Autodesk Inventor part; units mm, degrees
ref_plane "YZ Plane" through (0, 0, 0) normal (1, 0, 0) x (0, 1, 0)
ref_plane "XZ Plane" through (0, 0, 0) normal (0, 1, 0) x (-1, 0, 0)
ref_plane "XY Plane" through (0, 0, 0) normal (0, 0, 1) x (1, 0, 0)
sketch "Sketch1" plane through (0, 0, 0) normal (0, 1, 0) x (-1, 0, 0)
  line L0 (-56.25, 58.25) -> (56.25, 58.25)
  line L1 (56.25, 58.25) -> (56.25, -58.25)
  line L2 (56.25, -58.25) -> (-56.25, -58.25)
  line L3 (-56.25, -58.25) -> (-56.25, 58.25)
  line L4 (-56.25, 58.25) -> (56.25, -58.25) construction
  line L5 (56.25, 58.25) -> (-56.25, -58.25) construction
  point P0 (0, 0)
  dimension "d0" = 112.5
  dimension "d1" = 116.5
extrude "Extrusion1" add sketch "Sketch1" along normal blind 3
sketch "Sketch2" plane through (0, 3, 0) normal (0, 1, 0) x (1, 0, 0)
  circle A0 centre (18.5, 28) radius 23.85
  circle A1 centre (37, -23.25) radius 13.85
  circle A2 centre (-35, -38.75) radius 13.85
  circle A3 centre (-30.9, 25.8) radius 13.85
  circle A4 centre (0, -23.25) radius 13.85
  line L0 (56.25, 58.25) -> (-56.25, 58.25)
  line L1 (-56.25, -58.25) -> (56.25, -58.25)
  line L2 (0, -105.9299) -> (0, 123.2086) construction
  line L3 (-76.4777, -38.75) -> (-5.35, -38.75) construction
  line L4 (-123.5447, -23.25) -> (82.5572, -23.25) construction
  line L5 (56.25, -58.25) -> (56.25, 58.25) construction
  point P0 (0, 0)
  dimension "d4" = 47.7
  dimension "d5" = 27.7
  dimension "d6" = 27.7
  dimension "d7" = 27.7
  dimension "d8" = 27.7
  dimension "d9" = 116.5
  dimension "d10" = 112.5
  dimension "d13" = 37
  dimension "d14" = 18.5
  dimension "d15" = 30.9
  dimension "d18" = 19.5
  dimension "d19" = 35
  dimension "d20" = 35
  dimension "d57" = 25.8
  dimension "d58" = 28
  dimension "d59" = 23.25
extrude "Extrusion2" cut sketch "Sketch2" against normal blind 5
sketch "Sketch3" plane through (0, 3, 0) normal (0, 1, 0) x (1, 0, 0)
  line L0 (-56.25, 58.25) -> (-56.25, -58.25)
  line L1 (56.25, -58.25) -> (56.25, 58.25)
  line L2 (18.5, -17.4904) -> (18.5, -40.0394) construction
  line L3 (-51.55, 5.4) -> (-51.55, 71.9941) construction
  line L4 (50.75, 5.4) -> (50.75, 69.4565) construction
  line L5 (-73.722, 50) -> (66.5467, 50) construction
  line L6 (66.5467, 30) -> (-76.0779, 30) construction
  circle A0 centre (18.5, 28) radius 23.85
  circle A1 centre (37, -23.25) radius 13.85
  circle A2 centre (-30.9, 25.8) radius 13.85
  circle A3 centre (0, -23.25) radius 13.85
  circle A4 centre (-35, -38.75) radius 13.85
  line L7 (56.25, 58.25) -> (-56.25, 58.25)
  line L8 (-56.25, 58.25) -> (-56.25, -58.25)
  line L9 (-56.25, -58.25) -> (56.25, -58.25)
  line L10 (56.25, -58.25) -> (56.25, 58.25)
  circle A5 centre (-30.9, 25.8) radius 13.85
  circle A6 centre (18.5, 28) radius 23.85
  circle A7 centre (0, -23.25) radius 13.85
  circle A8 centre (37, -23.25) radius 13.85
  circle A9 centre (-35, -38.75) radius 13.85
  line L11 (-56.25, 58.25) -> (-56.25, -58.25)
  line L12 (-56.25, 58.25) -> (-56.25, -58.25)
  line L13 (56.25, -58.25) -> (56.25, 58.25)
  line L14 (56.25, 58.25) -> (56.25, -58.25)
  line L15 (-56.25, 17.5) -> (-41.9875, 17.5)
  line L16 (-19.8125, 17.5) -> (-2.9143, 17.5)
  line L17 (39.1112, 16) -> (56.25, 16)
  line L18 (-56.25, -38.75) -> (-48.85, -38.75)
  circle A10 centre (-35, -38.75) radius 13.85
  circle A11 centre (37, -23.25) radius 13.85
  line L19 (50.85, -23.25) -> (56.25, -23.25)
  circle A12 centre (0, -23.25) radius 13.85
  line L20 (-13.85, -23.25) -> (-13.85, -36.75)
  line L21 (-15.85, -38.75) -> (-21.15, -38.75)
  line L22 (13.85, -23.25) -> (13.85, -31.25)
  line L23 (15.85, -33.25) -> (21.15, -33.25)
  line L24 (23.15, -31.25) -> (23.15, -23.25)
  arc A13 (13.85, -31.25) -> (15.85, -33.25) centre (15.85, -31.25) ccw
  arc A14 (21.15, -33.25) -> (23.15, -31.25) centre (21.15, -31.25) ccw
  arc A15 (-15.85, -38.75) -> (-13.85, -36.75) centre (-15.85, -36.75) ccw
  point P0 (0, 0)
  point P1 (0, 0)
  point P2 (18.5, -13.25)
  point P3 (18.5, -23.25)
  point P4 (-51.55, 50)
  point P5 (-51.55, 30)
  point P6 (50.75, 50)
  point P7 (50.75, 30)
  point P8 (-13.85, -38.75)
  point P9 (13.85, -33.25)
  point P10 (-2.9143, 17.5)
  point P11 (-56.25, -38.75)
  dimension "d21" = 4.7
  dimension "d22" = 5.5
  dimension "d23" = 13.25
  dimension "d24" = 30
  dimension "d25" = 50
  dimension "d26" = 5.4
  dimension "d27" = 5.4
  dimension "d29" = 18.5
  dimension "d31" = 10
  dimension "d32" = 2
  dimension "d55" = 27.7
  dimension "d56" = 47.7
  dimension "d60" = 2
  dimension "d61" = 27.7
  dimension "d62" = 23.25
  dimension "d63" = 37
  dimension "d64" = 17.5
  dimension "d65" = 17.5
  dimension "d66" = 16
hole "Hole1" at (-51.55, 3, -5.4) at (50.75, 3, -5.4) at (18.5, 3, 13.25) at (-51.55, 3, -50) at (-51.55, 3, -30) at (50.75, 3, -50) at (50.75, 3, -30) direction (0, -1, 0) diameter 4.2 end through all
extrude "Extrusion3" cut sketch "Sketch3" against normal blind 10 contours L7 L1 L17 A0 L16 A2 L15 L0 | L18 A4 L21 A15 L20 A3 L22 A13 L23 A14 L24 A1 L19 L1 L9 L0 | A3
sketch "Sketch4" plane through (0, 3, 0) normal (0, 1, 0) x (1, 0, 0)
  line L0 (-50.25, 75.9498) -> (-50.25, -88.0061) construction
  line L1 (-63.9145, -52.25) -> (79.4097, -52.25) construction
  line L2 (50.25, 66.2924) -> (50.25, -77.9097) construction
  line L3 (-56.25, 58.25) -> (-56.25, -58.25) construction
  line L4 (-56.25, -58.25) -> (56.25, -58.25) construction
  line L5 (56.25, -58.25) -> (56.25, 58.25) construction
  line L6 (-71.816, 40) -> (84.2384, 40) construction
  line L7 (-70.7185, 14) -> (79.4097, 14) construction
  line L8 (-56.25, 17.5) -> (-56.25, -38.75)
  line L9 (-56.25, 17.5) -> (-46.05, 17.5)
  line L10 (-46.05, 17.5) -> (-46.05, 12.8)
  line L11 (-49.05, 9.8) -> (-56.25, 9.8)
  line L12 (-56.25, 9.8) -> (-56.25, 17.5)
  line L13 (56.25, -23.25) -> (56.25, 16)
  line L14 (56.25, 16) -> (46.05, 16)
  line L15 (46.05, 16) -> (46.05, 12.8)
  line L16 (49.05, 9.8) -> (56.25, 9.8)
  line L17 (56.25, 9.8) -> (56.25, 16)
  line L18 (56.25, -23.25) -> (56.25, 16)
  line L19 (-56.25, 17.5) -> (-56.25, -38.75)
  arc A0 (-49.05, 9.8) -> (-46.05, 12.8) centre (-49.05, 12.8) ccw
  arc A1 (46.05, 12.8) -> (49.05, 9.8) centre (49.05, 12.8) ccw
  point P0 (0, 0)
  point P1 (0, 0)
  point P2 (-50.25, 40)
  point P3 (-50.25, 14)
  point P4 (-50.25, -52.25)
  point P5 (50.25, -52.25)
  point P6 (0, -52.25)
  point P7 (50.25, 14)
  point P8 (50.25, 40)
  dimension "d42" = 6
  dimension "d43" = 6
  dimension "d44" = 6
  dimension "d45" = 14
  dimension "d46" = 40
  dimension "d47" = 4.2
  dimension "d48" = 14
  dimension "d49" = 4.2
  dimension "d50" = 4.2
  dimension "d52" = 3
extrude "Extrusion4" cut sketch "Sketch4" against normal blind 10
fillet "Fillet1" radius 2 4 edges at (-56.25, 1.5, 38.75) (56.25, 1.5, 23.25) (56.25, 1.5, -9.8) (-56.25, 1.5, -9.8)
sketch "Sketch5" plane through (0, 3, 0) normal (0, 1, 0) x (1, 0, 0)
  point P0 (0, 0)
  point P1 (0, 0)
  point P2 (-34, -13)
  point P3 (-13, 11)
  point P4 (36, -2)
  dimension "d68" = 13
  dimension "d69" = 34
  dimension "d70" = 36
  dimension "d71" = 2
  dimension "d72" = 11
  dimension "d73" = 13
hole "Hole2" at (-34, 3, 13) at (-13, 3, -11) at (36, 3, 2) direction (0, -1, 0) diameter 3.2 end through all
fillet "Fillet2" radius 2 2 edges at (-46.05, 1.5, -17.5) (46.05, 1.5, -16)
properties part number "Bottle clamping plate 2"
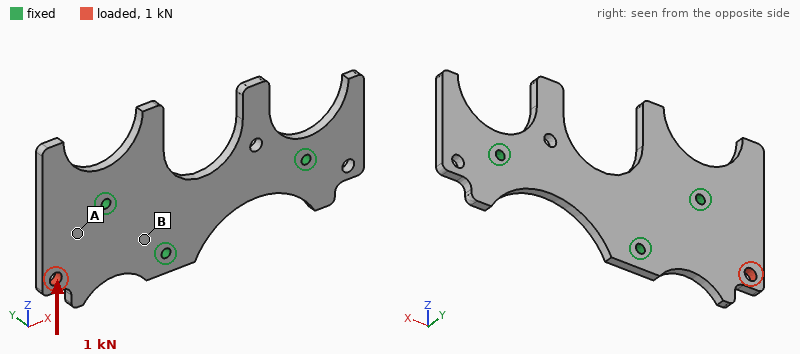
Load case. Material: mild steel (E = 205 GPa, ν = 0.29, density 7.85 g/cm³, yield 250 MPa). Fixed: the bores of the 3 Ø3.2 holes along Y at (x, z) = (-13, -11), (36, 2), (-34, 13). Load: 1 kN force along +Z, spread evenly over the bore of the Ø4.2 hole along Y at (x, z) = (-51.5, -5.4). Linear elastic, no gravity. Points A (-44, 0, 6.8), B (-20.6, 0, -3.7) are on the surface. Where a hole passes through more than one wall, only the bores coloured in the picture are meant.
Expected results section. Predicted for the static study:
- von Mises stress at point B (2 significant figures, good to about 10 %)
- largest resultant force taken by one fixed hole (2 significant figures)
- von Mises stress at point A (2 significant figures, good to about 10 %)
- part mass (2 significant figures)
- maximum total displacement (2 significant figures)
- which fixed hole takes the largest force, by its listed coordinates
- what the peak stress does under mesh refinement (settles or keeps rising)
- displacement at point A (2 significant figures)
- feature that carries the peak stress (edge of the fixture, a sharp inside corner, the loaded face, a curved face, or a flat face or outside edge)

10 MPa
1.3 kN
24 MPa
87 g
8.3 µm
(-34, 13)
keeps rising
3.1 µm
edge of the fixture
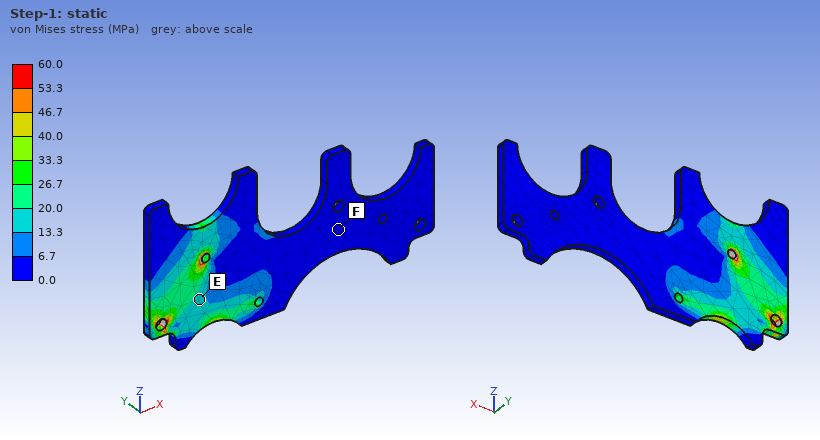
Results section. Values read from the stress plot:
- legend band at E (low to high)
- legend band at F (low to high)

13.3 to 20.0 MPa
0.0 to 6.7 MPa
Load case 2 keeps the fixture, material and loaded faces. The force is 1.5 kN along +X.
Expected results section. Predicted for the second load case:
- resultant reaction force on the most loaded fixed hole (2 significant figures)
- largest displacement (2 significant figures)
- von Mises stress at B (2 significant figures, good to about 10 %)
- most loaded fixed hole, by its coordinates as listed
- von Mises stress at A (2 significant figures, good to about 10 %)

930 N
9.0 µm
19 MPa
(-13, -11)
8.1 MPa
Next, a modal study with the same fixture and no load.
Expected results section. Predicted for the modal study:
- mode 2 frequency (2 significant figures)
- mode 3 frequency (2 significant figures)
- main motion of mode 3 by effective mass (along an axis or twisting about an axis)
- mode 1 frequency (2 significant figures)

3300 Hz
3400 Hz
twisting about X
2600 Hz
